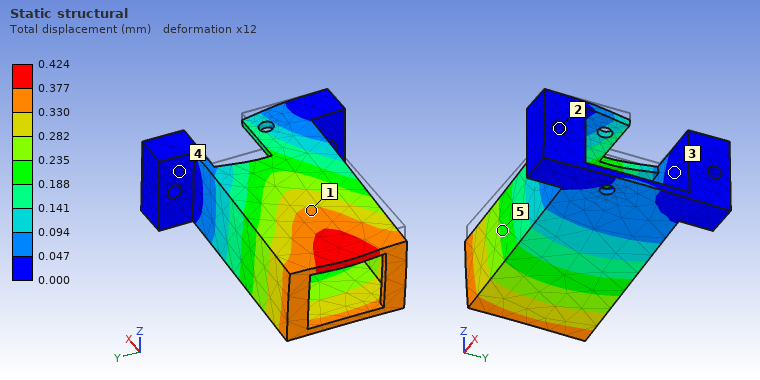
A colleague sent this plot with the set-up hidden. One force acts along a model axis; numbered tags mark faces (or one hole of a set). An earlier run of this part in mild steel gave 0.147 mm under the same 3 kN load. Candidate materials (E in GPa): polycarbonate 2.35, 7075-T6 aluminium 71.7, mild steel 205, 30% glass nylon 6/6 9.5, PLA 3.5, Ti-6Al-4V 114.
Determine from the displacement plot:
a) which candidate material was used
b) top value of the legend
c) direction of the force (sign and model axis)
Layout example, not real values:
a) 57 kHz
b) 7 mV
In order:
a) 7075-T6 aluminium
b) 0.424 mm
c) -Z
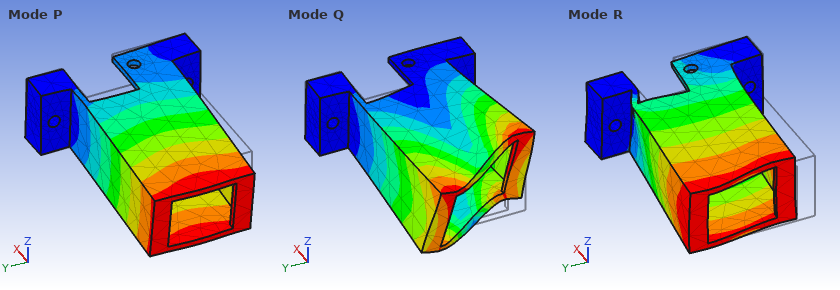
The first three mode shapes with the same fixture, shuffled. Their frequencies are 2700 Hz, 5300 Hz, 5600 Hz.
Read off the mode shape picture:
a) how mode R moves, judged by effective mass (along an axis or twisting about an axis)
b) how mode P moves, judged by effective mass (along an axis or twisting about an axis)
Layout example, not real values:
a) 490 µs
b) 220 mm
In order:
a) along Y
b) along Z
